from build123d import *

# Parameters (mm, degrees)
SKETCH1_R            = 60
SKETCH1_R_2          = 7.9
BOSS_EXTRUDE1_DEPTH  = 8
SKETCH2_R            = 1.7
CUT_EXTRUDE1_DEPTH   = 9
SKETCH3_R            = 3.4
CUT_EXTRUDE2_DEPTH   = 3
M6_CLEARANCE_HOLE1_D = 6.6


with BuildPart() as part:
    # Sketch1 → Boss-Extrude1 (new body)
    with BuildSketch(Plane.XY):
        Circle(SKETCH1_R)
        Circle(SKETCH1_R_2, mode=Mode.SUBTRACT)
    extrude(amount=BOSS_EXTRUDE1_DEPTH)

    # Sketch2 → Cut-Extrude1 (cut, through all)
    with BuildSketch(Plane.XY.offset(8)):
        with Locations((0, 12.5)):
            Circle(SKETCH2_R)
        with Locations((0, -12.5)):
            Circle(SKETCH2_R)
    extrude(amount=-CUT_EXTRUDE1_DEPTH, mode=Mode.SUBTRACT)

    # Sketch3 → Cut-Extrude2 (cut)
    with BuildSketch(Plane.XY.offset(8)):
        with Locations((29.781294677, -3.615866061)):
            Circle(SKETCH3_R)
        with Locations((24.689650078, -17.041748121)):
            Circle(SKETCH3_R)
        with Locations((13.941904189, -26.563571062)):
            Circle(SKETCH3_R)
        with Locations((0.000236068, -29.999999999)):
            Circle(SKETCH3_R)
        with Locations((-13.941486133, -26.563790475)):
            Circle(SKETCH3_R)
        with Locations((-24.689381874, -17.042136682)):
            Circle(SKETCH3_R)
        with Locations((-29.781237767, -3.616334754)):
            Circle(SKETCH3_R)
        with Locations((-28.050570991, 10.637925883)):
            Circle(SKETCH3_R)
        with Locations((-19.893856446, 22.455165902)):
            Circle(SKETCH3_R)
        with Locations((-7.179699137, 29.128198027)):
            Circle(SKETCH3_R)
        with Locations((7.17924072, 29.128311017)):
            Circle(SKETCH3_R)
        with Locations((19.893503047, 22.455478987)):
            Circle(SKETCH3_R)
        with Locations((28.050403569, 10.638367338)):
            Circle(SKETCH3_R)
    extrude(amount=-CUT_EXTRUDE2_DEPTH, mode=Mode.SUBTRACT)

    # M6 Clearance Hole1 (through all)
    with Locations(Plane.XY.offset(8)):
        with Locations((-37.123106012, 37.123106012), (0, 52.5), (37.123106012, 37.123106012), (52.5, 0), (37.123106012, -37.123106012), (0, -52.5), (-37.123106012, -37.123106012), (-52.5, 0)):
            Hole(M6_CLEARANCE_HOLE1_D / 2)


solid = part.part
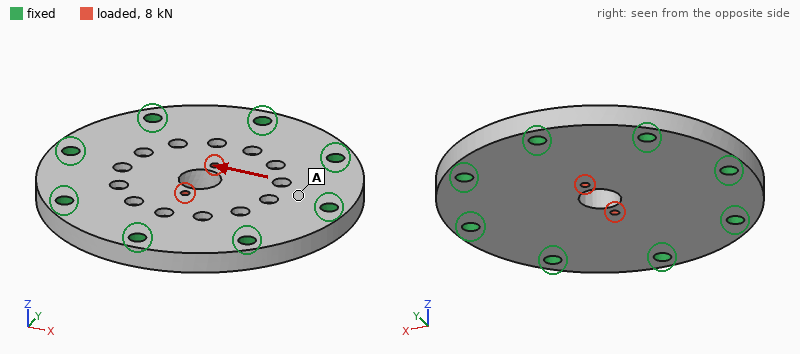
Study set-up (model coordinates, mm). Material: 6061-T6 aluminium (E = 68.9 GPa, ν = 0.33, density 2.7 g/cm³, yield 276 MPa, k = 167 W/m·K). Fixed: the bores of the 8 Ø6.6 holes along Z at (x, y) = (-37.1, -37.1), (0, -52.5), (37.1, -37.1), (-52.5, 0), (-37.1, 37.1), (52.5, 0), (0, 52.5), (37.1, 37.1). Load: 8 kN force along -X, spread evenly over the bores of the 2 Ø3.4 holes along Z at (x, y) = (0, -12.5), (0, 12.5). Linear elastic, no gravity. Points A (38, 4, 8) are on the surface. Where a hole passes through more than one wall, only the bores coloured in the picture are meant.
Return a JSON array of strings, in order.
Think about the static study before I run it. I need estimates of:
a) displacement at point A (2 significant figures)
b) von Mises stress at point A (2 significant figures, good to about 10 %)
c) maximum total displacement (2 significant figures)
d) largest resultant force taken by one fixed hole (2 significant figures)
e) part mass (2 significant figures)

["1.8 µm", "8.4 MPa", "9.0 µm", "1.5 kN", "230 g"]
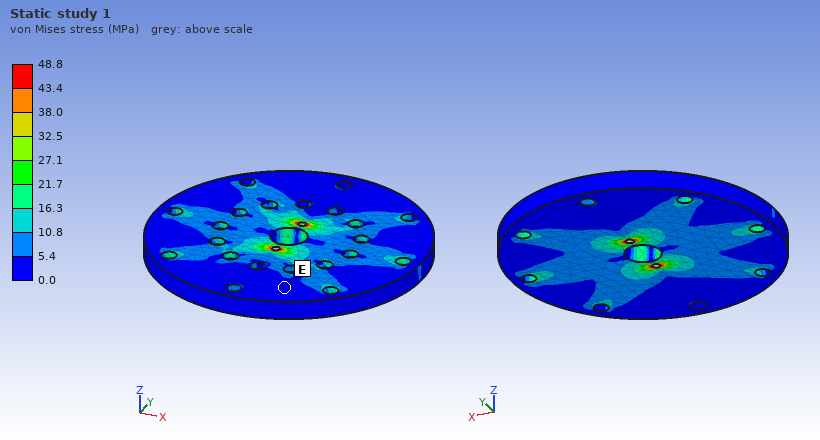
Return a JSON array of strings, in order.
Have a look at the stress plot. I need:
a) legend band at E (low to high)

["0.0 to 5.4 MPa"]
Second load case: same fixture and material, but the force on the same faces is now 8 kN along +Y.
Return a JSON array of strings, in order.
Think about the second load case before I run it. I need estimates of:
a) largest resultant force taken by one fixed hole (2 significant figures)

["1.8 kN"]
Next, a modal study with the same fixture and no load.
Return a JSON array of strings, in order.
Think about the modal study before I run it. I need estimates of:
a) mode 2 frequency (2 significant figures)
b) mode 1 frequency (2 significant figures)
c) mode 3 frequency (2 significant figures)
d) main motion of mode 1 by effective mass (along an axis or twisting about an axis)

["12 kHz", "6200 Hz", "12 kHz", "along Z"]
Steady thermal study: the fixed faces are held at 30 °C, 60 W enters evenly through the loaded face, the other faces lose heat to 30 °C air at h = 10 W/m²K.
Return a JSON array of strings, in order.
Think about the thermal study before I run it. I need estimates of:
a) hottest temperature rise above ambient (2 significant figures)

["18 K"]
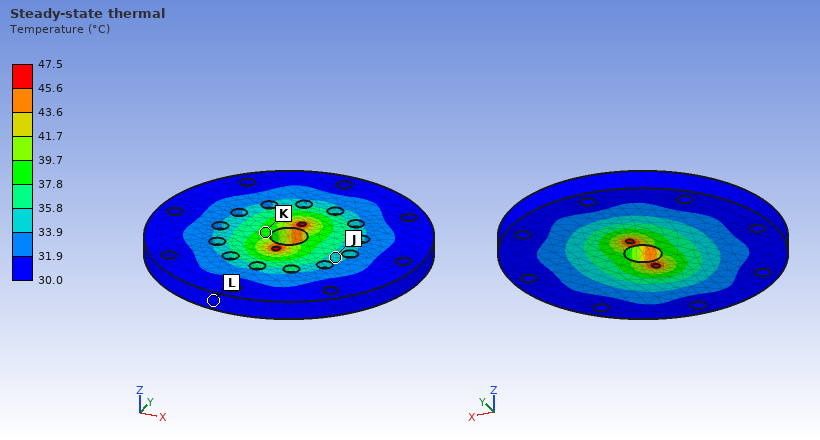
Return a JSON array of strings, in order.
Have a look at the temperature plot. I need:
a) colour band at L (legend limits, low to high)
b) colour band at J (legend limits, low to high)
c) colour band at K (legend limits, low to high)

["30.0 to 31.9 °C", "33.9 to 35.8 °C", "37.8 to 39.7 °C"]
